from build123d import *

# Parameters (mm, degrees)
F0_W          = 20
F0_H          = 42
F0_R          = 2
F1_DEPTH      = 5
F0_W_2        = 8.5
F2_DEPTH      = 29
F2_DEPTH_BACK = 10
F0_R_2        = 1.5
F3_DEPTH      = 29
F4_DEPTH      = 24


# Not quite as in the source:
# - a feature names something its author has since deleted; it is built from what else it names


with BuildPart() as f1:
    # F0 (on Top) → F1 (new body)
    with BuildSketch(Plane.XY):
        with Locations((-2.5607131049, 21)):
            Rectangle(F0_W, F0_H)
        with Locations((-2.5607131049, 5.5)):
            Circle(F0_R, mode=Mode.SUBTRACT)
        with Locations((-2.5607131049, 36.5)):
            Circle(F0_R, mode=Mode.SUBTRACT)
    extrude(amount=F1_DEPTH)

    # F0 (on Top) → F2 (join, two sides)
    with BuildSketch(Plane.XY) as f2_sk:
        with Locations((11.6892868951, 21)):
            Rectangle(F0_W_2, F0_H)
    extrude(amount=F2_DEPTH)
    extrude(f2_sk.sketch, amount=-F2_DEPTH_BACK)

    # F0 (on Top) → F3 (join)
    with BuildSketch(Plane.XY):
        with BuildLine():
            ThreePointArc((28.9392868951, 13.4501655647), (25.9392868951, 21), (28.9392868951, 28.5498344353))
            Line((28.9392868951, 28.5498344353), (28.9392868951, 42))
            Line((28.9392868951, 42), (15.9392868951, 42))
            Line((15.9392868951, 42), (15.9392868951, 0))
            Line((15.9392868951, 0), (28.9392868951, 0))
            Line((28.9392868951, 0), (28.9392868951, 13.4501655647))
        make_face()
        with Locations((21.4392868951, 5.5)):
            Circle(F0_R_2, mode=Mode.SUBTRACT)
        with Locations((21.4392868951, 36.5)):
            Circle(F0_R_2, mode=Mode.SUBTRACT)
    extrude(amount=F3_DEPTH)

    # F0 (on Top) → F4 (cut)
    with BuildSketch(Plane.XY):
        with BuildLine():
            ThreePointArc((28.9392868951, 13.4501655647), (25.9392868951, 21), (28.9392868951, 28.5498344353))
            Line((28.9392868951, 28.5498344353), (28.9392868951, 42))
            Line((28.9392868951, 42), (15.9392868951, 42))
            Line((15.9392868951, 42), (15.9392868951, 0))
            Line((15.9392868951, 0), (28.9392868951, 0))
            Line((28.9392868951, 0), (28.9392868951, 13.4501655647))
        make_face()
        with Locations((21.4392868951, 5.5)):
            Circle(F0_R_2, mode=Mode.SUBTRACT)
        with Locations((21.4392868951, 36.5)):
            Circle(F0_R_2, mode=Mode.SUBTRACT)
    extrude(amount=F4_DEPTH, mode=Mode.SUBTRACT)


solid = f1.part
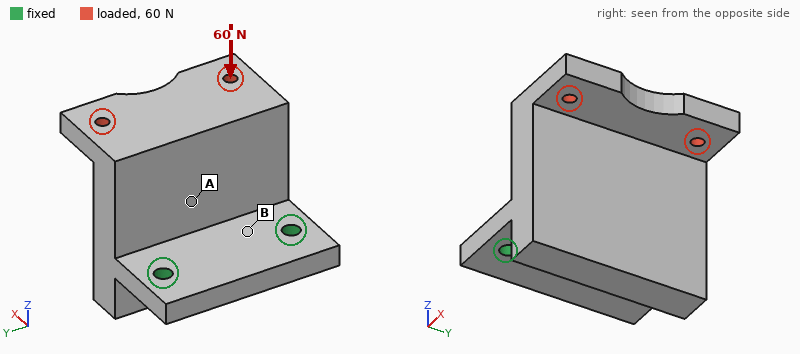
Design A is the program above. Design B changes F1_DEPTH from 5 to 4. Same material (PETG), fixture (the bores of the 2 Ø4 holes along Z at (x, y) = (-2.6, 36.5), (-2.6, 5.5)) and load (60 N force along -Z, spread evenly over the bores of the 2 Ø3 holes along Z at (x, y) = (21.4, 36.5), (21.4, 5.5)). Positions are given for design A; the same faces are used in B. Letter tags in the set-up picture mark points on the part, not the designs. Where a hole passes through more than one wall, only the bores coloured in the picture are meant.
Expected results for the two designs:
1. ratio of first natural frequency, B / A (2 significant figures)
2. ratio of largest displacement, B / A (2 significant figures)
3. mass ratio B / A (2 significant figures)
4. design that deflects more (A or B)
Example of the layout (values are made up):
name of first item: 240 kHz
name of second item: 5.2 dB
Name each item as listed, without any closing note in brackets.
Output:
ratio of first natural frequency, B / A: 0.74
ratio of largest displacement, B / A: 1.7
mass ratio B / A: 0.96
design that deflects more: B
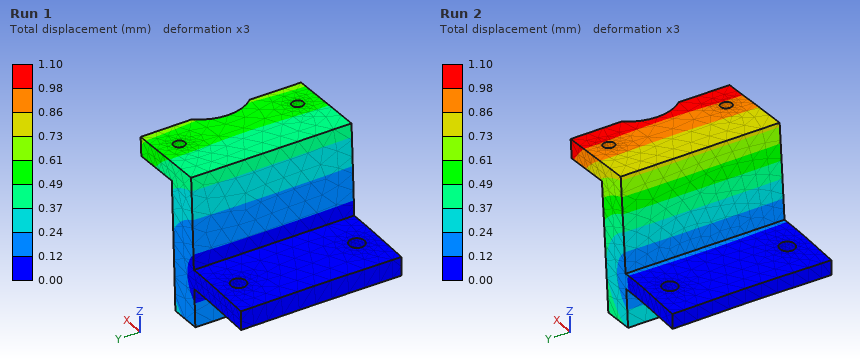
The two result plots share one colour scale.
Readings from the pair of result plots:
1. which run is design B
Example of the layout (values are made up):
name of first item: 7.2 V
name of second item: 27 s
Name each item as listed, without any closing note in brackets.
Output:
which run is design B: Run 2
